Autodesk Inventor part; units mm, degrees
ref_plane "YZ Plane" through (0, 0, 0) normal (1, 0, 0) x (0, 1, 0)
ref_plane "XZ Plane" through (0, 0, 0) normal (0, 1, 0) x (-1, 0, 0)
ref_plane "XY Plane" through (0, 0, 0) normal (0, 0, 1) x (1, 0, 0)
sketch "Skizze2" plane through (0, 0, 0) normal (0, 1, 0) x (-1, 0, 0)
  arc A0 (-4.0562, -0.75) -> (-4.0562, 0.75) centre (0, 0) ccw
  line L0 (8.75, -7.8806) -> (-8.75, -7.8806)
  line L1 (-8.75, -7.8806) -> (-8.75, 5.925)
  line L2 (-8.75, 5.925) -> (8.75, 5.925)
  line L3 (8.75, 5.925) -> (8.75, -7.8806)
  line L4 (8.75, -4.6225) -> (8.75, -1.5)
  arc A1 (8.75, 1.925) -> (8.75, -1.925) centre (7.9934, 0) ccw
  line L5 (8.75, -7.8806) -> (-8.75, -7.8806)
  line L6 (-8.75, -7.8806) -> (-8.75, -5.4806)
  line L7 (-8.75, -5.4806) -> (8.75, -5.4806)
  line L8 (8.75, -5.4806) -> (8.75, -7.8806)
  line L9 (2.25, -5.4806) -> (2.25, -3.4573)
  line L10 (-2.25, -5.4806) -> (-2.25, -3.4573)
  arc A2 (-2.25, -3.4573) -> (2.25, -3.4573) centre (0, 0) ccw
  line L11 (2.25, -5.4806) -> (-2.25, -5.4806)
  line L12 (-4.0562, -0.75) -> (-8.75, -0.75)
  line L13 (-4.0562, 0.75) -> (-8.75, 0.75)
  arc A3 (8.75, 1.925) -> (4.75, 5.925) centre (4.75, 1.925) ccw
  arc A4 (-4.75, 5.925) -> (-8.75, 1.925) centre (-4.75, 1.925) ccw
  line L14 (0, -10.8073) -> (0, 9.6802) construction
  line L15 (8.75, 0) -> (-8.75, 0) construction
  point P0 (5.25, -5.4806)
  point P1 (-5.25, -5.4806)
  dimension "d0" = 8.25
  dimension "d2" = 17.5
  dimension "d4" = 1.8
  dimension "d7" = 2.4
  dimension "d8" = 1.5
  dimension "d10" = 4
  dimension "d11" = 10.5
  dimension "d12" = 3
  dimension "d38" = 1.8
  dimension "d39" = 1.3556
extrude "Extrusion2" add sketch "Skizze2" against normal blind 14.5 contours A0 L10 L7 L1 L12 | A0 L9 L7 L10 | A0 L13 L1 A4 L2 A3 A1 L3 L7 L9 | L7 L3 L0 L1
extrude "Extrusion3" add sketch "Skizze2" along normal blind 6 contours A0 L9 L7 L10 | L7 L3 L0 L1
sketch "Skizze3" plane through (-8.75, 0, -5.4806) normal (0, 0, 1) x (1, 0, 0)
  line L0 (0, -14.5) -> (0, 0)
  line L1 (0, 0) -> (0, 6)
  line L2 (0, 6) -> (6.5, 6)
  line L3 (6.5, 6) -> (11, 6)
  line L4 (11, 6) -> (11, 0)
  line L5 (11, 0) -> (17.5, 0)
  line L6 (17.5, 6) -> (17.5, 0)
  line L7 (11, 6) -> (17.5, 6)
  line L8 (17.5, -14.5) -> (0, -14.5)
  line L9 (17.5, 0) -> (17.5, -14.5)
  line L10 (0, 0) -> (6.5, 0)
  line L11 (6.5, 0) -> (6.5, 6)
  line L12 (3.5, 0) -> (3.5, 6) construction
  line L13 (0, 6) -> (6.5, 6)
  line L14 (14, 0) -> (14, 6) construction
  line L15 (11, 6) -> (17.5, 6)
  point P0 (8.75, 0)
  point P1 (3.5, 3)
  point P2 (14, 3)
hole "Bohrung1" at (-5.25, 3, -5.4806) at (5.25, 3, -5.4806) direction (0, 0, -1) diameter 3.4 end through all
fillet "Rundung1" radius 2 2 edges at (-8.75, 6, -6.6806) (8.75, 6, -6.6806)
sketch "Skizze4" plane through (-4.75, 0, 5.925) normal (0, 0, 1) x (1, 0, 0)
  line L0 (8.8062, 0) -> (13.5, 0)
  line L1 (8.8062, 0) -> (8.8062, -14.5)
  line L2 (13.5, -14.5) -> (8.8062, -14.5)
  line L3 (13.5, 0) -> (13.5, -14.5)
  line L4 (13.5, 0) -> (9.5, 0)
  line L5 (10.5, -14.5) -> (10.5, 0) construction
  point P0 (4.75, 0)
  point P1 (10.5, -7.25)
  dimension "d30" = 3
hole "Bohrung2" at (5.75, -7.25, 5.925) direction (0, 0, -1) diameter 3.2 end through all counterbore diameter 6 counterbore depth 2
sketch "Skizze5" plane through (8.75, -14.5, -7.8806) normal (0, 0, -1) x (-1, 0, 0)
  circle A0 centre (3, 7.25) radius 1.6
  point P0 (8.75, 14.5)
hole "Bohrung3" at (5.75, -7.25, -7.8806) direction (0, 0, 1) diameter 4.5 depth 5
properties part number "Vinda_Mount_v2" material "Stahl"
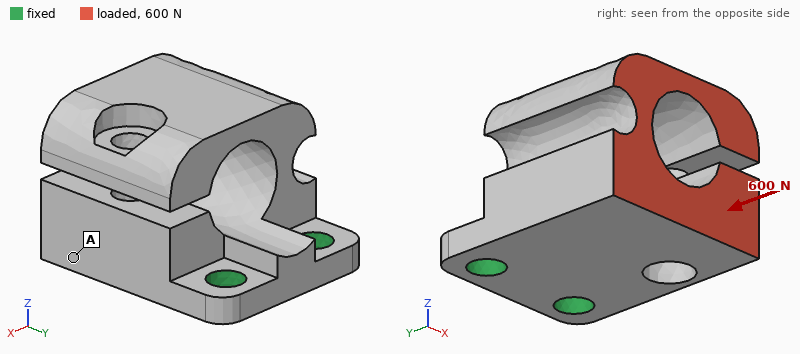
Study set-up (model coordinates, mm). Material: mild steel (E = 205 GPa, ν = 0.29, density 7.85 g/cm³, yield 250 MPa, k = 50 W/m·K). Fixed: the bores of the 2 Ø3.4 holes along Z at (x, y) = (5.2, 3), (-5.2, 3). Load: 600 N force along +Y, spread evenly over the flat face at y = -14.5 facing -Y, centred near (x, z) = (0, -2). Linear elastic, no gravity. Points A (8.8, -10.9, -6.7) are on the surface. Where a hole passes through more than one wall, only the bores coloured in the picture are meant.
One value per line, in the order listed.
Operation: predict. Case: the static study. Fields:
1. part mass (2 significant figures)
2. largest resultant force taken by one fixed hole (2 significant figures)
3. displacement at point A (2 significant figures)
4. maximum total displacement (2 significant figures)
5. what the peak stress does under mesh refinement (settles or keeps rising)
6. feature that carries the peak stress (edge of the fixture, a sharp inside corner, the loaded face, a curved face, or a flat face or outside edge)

19 g
310 N
18 µm
43 µm
keeps rising
edge of the fixture
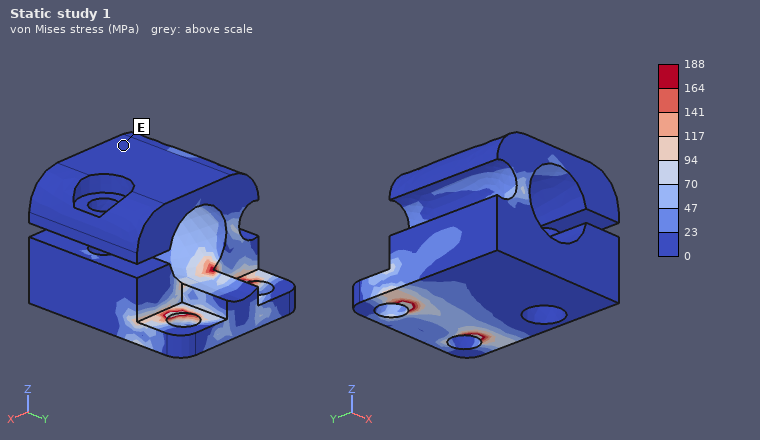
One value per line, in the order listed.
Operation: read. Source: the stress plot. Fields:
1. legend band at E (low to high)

0 to 23 MPa
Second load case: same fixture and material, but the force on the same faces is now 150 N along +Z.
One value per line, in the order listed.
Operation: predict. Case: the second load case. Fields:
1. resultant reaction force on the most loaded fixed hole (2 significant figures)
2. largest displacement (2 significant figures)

85 N
40 µm
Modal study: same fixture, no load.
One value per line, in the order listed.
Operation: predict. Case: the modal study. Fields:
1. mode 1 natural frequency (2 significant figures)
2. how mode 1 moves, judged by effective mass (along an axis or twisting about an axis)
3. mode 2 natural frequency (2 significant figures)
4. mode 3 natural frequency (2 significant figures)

3900 Hz
along Z
5100 Hz
9900 Hz
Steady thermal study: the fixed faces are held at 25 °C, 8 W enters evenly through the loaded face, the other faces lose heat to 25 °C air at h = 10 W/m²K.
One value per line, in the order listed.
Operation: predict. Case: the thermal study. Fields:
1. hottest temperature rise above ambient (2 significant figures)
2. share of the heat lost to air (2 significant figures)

48 K
5.9 %
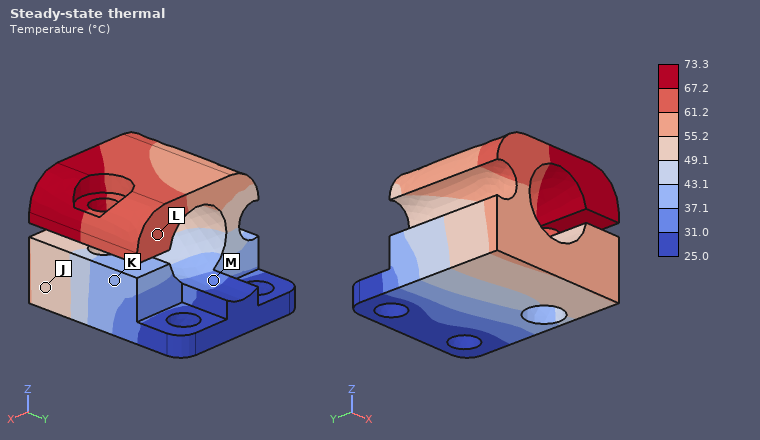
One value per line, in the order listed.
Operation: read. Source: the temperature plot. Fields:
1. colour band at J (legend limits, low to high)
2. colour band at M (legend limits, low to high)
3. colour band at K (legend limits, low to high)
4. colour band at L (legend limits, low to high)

49.1 to 55.2 °C
31.0 to 37.1 °C
37.1 to 43.1 °C
61.2 to 67.2 °C
